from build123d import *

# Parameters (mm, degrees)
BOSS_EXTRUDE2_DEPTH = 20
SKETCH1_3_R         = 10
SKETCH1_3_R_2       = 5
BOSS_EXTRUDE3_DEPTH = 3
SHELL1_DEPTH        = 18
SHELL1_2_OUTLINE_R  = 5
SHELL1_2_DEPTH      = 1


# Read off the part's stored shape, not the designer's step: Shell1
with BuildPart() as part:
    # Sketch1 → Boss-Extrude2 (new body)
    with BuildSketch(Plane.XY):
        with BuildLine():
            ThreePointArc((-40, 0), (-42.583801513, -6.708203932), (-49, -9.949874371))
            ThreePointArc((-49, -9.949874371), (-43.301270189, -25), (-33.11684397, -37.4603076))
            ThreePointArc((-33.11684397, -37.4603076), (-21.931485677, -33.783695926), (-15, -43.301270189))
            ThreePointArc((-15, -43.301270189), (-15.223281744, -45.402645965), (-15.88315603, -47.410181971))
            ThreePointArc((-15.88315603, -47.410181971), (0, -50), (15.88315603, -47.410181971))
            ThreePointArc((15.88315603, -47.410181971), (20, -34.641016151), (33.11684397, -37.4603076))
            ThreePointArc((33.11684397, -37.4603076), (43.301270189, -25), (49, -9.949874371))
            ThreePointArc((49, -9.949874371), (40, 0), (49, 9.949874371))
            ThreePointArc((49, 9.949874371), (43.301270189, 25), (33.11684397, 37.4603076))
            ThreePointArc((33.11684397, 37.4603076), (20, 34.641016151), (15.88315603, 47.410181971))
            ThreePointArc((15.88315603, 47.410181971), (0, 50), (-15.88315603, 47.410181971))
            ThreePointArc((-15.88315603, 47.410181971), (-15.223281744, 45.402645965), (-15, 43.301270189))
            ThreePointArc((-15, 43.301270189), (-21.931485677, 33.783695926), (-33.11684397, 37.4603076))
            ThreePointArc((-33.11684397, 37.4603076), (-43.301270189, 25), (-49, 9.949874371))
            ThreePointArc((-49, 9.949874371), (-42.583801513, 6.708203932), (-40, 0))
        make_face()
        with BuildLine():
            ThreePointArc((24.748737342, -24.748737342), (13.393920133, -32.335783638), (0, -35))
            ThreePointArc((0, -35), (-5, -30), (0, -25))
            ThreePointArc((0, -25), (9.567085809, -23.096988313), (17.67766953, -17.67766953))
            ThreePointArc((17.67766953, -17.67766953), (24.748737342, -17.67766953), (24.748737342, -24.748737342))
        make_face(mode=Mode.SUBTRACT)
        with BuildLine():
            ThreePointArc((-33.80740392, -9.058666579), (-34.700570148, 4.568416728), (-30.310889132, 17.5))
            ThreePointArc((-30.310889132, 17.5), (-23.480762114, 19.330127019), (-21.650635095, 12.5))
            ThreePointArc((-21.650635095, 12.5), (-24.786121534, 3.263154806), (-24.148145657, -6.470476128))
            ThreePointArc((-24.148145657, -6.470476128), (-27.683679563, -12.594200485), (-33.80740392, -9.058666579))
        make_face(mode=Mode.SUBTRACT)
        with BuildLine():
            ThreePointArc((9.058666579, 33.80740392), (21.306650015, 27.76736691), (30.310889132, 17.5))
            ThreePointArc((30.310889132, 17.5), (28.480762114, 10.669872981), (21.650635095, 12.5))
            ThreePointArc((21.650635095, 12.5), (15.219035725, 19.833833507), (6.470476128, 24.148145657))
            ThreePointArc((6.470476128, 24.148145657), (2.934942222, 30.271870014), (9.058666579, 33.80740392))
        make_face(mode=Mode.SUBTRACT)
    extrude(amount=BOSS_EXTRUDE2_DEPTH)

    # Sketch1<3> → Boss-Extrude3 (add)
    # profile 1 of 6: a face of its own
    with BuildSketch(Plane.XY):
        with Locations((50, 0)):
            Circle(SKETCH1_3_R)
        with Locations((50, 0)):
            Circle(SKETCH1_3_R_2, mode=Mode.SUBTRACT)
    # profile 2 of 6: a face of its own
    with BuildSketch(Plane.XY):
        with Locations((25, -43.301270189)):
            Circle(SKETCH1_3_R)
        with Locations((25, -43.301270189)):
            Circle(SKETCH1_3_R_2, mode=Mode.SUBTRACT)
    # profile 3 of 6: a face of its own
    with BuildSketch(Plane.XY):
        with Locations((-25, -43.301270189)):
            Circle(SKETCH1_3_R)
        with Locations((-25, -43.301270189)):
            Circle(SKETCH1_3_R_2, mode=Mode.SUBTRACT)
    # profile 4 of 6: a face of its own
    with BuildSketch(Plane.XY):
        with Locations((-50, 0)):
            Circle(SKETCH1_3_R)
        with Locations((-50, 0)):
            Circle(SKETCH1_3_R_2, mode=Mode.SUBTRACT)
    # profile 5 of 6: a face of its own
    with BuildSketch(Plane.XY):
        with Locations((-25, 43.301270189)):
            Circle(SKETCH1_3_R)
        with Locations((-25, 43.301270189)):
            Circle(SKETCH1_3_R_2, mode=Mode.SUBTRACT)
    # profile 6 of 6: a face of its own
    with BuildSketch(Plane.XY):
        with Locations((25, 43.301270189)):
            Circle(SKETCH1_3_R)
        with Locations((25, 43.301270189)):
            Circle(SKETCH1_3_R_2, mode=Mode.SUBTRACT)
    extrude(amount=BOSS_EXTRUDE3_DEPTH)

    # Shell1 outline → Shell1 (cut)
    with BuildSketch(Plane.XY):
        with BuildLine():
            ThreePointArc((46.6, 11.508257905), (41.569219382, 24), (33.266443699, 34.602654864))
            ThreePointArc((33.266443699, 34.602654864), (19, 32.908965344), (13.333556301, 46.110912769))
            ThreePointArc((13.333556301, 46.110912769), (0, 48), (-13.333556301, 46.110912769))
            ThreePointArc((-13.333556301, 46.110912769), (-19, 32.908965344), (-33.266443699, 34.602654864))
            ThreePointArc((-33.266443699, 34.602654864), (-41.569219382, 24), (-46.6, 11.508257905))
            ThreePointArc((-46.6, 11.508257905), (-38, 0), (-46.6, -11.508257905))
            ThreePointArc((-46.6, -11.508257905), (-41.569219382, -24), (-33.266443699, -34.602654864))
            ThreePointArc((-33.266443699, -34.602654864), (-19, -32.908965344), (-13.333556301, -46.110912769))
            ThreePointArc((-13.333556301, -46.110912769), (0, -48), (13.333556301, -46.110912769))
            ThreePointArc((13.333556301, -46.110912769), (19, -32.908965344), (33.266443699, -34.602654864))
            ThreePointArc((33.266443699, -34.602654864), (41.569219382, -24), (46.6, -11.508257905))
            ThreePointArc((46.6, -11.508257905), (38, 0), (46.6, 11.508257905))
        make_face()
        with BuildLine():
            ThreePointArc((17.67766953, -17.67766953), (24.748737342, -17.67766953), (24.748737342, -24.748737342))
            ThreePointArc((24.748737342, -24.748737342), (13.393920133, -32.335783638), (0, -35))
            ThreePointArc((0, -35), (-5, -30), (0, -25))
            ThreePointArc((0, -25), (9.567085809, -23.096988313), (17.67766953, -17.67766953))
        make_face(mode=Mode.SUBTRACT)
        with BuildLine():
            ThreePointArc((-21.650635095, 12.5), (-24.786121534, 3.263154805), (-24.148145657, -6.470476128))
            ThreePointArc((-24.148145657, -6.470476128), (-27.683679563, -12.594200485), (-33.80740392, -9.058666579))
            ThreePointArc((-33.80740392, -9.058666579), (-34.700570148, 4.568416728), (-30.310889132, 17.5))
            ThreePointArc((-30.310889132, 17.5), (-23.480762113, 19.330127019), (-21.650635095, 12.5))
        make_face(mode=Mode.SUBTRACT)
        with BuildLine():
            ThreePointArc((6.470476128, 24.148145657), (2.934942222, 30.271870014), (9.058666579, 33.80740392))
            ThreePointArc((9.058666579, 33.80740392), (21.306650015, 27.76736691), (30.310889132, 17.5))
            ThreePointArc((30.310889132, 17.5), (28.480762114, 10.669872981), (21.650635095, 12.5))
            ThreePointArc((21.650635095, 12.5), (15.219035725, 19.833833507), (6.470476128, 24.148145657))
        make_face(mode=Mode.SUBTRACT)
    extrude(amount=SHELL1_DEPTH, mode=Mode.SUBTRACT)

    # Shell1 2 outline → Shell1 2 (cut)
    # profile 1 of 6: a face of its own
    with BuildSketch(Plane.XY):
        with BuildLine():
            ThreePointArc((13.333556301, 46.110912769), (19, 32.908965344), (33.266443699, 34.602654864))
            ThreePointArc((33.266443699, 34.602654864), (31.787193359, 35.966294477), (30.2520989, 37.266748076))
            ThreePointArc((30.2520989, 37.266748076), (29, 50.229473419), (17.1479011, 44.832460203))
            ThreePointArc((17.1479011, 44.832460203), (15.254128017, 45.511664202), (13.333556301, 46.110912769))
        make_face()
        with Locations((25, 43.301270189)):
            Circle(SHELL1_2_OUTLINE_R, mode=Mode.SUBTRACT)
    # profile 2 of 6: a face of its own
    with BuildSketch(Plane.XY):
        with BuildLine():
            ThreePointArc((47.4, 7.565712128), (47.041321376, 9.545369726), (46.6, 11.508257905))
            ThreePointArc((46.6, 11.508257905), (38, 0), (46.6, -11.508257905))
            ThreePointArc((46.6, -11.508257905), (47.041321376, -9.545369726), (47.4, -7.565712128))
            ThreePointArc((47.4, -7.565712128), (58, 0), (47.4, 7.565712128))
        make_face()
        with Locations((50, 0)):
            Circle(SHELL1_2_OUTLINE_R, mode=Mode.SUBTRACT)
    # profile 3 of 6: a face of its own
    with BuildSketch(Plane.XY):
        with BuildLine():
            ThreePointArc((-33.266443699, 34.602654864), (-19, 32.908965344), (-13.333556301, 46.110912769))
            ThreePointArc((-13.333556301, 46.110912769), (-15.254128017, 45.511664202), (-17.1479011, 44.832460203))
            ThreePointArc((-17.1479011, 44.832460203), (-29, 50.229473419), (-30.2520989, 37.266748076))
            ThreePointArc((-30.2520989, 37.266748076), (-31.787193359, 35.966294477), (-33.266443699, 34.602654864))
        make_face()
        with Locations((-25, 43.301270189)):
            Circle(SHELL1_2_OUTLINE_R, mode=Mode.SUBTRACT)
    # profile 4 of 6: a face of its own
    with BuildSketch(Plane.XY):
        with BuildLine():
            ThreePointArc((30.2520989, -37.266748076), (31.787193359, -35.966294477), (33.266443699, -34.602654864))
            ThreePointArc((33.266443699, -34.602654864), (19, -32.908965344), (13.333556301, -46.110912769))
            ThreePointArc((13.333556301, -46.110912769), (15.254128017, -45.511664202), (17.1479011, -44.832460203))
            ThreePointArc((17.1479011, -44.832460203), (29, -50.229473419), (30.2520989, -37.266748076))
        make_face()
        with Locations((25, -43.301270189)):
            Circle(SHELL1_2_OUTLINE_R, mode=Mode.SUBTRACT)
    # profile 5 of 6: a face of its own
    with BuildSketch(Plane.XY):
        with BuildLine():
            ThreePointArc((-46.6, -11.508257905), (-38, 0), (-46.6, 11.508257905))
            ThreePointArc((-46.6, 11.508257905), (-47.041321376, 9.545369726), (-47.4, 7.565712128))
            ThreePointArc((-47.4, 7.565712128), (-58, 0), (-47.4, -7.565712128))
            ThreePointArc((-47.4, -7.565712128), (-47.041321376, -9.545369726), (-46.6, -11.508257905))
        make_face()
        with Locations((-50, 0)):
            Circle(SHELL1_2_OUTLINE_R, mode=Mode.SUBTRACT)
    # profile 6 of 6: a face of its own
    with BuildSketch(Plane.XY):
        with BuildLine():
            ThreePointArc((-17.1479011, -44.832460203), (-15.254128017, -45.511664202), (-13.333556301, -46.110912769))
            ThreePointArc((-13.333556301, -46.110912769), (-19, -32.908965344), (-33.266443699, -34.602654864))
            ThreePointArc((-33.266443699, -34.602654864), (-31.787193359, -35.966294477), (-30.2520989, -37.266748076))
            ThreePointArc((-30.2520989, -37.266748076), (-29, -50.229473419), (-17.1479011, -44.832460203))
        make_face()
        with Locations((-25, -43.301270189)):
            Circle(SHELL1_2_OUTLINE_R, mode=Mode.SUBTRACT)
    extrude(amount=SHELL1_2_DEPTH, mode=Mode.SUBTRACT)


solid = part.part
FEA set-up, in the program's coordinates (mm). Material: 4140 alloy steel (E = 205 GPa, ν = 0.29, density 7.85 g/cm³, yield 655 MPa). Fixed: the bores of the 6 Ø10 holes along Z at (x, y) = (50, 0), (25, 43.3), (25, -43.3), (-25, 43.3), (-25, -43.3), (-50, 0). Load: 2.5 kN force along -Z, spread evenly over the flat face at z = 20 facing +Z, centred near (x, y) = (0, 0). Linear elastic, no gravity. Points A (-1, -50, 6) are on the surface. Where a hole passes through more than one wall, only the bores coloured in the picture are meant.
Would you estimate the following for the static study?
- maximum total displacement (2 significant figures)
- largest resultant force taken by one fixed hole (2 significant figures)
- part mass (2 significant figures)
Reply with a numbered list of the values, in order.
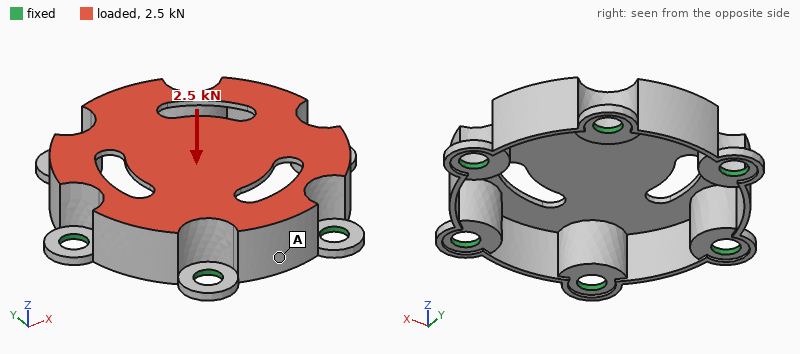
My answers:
1. 0.19 mm
2. 570 N
3. 220 g
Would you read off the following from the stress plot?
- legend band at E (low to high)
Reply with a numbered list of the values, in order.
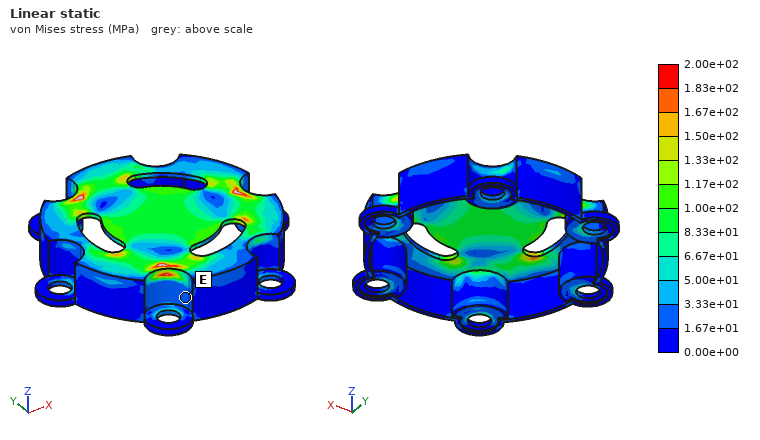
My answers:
1. 1.67e+01 to 3.33e+01 MPa
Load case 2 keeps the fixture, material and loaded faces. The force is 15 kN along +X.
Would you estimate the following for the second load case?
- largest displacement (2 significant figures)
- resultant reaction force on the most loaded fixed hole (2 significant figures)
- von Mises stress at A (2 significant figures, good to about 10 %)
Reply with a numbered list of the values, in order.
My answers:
1. 92 µm
2. 4.1 kN
3. 52 MPa
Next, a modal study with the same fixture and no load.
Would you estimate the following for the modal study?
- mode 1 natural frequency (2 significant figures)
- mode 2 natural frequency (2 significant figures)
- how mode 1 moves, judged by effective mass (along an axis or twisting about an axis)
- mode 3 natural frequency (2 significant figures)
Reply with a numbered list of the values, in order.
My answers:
1. 2200 Hz
2. 4300 Hz
3. along Z
4. 4300 Hz
